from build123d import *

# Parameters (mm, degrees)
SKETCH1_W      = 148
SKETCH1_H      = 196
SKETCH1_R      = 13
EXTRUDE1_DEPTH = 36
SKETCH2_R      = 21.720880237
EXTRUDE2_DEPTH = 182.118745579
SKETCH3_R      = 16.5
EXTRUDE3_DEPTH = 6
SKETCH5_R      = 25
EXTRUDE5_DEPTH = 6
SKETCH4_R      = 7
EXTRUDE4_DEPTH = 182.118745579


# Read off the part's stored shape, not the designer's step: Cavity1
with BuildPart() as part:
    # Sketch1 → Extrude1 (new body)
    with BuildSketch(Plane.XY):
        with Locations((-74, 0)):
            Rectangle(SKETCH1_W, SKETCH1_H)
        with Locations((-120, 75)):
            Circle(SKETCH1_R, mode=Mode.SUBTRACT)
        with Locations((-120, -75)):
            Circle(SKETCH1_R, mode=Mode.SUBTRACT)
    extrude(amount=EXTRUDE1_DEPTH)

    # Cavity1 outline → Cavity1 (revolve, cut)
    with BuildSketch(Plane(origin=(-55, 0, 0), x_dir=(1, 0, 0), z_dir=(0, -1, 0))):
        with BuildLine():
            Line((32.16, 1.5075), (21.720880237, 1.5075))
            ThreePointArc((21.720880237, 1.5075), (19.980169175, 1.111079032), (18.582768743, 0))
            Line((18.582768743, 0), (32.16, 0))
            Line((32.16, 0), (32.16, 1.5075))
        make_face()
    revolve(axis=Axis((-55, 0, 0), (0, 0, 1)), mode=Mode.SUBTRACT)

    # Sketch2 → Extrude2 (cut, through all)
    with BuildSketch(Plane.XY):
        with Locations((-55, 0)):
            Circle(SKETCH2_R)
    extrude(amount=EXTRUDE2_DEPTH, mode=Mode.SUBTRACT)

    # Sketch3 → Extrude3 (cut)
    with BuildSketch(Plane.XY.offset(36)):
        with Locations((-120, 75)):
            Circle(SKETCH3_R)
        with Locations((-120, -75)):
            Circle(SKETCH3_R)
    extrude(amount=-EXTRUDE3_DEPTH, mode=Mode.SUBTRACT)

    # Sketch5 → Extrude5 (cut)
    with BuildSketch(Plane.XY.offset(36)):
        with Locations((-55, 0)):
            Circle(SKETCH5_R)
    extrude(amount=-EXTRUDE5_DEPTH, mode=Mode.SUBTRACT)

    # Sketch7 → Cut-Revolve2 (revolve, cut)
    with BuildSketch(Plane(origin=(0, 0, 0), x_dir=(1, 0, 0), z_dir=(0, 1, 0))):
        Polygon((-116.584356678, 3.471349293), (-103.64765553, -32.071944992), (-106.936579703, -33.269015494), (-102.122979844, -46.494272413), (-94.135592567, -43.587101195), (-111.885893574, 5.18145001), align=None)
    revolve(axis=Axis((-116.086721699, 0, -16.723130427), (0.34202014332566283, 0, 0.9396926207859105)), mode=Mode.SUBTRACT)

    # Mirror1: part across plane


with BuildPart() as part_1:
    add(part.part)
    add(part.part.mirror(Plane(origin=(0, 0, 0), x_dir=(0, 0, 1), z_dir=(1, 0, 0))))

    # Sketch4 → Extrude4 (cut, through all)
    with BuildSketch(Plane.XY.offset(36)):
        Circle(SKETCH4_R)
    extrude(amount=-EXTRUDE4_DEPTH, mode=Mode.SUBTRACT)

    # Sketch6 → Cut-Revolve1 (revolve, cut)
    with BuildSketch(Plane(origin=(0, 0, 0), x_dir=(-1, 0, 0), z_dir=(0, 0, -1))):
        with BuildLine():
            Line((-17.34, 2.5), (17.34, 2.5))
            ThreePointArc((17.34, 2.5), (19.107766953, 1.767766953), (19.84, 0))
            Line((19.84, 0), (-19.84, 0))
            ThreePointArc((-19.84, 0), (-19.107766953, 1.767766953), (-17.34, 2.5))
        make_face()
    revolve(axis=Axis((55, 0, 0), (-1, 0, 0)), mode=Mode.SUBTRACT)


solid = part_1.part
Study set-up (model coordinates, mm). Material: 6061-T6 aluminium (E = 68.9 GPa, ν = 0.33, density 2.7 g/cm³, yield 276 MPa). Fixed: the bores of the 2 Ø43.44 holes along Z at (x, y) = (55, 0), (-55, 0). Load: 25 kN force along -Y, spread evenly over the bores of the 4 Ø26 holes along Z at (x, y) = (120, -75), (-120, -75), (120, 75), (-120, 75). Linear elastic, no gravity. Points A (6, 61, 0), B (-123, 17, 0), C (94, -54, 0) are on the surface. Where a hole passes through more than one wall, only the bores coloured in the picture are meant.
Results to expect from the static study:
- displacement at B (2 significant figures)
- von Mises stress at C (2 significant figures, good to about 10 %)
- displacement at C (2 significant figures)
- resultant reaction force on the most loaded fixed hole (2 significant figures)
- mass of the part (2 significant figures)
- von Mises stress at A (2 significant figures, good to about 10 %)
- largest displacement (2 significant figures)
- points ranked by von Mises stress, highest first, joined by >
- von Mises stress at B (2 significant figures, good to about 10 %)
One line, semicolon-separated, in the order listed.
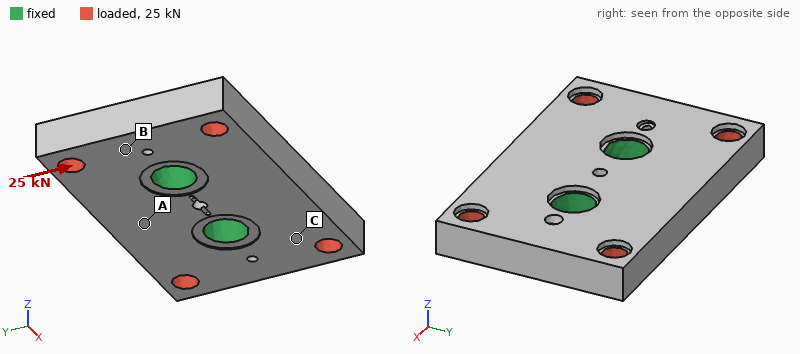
6.9 µm; 4.8 MPa; 5.0 µm; 13 kN; 5.1 kg; 1.3 MPa; 13 µm; C > B > A; 2.3 MPa
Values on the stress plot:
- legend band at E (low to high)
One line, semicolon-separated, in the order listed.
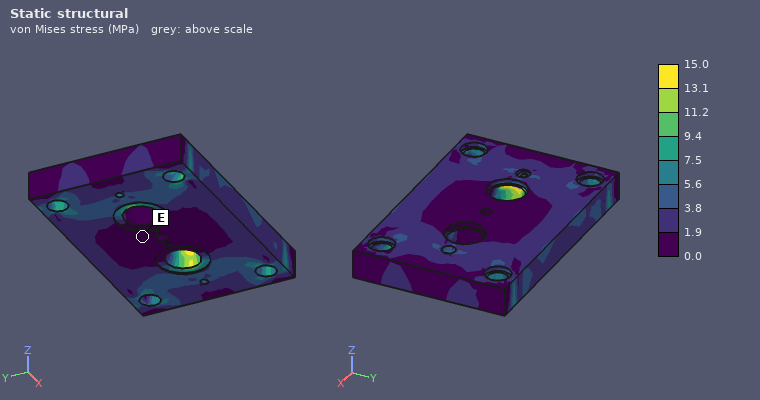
0.0 to 1.9 MPa
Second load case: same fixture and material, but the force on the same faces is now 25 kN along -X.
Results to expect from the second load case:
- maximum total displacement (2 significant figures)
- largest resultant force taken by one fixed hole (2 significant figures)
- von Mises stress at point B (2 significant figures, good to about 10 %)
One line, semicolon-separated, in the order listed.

9.1 µm; 13 kN; 1.7 MPa
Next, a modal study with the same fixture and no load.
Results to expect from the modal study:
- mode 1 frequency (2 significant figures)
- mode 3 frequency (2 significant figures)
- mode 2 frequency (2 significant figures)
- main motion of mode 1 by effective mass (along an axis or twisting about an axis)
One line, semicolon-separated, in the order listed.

2500 Hz; 2800 Hz; 2700 Hz; twisting about X
